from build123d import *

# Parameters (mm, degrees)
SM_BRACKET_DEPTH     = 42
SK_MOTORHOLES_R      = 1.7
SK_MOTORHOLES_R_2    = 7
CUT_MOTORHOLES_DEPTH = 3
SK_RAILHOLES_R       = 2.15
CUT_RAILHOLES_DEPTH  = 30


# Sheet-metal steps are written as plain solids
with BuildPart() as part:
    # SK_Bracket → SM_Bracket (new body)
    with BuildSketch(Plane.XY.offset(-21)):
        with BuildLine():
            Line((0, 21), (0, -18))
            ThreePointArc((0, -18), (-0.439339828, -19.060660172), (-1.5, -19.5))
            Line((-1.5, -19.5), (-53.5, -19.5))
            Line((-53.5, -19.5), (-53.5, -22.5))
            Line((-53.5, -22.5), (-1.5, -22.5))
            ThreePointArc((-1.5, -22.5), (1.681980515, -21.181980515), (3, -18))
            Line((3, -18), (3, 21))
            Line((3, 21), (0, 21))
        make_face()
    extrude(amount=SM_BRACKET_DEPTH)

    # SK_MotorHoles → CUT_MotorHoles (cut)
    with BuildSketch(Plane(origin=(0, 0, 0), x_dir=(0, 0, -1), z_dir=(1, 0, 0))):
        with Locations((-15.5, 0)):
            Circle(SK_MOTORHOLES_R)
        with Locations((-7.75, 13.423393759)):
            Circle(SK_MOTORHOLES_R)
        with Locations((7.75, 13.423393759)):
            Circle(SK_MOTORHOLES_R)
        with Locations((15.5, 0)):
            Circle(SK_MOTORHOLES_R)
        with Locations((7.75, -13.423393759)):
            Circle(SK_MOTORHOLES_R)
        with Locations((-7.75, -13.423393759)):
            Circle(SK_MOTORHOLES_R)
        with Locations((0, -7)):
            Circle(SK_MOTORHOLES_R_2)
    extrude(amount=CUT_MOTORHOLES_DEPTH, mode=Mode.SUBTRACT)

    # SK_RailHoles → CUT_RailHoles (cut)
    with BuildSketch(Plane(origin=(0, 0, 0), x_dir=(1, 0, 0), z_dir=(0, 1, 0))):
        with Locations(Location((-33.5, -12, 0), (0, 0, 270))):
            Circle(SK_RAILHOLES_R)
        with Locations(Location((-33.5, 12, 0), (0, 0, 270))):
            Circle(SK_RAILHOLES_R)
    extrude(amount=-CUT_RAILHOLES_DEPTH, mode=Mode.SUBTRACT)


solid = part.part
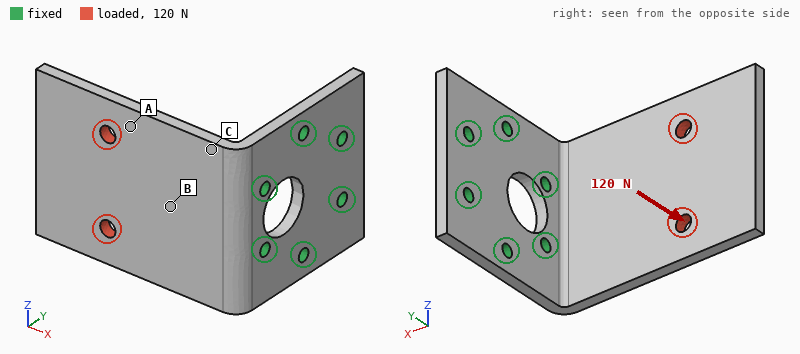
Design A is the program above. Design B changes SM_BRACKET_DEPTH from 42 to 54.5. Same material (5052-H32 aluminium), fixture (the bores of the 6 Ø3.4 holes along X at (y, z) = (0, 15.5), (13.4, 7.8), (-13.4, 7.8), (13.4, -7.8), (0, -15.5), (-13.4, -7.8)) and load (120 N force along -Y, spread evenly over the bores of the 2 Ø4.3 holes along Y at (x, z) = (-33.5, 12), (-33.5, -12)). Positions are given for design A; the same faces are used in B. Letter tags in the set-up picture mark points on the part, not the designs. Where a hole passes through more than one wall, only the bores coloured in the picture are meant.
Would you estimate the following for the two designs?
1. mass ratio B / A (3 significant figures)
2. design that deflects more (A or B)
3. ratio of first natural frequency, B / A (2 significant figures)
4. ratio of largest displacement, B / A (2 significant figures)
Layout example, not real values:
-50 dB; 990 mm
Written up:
1.32; A; 0.98; 0.84
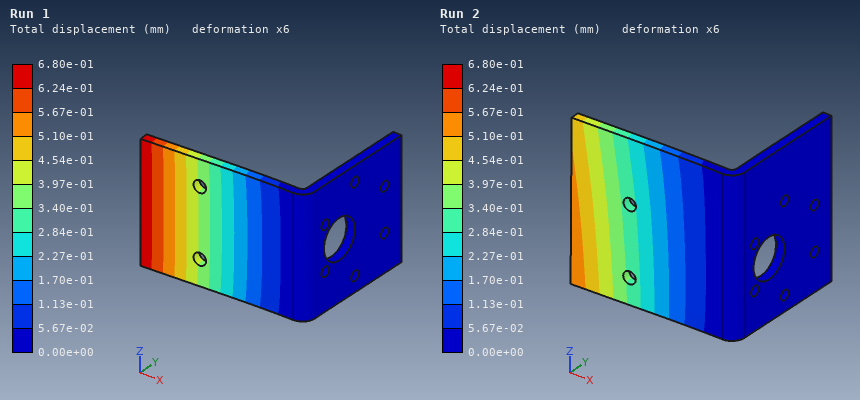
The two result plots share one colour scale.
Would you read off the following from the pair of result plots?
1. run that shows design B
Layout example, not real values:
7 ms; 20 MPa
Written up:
Run 2
